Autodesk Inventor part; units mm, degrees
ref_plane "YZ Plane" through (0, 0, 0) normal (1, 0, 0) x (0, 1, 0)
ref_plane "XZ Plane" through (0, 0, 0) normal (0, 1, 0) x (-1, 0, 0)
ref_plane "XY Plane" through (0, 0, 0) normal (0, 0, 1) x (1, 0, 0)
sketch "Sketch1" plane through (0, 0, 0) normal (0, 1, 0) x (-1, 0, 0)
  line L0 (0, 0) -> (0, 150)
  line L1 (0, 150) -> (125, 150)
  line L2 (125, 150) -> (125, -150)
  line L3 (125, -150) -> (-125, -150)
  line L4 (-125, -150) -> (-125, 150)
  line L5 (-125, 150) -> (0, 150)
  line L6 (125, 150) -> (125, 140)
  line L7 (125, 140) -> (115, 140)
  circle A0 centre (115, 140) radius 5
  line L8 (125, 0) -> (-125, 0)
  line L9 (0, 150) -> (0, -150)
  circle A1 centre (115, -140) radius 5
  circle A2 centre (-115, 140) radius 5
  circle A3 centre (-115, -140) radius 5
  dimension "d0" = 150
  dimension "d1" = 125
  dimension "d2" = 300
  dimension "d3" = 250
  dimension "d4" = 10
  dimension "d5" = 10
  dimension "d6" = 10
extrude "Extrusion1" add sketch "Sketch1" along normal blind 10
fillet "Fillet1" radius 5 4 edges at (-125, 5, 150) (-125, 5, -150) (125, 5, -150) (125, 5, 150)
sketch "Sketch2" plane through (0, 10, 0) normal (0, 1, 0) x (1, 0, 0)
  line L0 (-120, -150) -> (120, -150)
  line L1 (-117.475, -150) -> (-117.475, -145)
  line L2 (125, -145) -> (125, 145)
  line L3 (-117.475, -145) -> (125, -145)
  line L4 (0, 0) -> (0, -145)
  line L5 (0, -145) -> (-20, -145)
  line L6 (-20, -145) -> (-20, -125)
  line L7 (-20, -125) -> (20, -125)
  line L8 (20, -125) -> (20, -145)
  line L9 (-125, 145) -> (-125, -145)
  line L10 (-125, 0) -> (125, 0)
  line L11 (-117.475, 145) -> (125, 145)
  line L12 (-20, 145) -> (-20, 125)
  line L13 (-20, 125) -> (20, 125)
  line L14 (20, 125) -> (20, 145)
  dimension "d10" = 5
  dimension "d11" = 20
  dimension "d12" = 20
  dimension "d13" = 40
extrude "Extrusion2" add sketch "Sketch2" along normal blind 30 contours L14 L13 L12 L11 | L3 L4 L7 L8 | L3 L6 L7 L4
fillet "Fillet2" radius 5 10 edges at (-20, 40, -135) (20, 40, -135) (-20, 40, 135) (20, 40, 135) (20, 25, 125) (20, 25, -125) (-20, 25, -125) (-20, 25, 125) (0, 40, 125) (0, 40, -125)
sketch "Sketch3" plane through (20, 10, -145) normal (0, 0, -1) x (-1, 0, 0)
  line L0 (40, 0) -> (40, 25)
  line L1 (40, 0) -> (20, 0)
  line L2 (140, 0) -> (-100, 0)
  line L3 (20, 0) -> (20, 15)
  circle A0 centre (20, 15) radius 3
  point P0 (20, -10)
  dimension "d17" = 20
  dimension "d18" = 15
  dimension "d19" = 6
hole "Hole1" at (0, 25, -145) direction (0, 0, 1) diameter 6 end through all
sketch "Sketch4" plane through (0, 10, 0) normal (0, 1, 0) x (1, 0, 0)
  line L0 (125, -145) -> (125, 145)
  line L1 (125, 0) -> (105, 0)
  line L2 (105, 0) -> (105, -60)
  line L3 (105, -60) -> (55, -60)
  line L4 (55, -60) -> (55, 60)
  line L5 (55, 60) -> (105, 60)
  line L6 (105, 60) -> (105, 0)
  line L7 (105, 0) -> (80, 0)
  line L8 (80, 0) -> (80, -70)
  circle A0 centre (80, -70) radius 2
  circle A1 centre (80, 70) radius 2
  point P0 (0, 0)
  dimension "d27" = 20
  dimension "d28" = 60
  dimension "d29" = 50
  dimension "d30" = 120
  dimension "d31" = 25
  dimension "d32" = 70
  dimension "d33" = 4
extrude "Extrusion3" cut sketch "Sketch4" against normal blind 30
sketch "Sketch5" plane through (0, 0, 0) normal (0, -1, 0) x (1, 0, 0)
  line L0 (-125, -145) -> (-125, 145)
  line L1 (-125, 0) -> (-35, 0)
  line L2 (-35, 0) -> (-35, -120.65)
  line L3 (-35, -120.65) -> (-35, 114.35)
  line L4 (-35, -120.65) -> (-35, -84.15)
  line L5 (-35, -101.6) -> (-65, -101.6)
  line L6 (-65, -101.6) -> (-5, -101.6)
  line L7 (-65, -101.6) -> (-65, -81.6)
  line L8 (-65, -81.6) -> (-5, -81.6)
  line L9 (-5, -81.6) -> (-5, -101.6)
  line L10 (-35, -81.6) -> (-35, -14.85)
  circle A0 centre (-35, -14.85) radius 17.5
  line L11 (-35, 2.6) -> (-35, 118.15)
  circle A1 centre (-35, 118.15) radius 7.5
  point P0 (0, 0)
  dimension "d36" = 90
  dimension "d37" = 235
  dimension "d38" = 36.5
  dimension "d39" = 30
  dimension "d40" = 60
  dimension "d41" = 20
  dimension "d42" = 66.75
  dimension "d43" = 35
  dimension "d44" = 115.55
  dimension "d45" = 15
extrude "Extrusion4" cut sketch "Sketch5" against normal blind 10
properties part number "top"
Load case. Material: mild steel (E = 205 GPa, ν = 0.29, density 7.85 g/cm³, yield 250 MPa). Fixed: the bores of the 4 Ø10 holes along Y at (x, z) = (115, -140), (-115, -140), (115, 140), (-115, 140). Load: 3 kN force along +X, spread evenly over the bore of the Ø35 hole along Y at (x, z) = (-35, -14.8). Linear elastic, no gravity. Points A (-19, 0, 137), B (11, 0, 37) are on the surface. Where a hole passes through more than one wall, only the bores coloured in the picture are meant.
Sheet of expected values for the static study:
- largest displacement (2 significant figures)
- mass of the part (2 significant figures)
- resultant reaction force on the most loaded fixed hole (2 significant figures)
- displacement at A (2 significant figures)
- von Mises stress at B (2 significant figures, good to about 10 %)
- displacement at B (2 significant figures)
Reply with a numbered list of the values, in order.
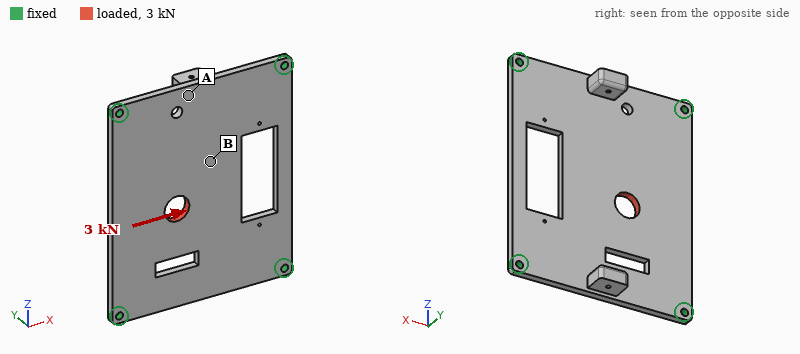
1. 2.4 µm
2. 5.6 kg
3. 950 N
4. 0.52 µm
5. 1.9 MPa
6. 1.5 µm
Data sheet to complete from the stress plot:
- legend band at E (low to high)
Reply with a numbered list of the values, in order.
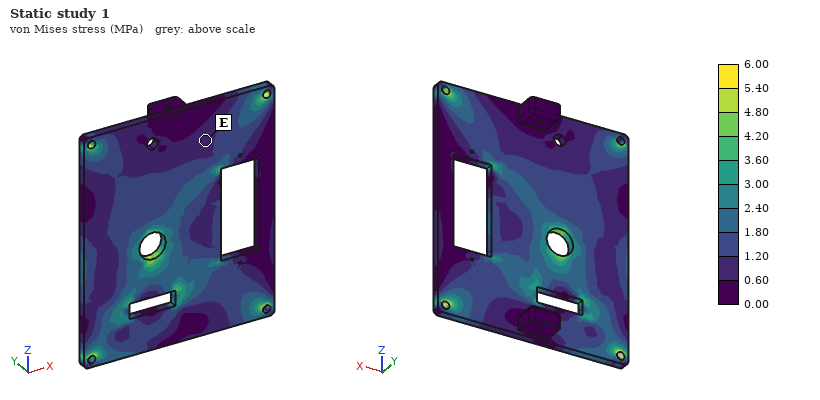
1. 0.60 to 1.20 MPa
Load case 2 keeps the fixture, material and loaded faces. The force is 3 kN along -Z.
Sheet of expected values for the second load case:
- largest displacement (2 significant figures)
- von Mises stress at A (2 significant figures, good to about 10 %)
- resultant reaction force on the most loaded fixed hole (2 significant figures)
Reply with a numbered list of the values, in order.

1. 1.9 µm
2. 0.52 MPa
3. 1.1 kN
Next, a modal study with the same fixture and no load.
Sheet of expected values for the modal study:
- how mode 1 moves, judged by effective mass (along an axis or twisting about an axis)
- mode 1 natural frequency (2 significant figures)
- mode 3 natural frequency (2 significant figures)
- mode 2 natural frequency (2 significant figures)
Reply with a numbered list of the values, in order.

1. along Y
2. 450 Hz
3. 850 Hz
4. 820 Hz
